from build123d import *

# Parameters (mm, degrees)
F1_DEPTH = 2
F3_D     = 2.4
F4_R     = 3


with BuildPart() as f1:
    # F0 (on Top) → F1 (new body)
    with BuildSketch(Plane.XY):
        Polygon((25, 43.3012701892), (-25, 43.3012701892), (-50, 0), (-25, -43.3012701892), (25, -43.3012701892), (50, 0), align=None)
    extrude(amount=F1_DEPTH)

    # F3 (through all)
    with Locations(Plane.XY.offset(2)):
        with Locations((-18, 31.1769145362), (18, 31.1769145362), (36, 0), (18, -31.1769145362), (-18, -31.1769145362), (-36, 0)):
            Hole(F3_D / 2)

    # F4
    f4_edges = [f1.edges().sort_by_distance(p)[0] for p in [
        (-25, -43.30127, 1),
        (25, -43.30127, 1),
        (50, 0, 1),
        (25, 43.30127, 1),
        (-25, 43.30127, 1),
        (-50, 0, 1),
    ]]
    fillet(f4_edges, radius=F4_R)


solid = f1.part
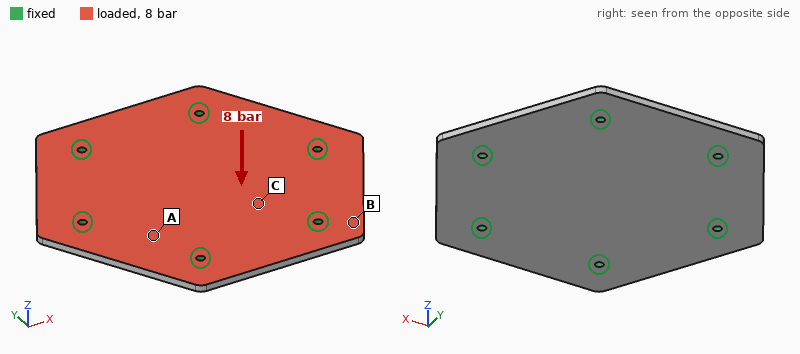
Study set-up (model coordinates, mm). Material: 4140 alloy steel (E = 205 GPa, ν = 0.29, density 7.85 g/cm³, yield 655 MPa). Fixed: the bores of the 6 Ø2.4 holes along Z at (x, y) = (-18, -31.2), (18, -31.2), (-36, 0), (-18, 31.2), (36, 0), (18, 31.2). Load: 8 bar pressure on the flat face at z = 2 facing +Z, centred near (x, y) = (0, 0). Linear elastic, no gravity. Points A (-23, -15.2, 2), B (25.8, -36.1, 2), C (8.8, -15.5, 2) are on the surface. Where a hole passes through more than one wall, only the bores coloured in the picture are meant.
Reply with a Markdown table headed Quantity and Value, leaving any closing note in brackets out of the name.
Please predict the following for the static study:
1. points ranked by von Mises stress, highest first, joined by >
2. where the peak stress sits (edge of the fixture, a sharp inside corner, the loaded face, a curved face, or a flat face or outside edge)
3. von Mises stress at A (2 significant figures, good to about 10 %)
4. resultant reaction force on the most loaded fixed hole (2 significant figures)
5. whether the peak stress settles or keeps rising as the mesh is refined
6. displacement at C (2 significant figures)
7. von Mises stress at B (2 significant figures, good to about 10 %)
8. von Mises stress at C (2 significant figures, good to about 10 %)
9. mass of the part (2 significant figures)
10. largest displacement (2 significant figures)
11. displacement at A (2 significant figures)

| Quantity | Value |
|---|---|
| points ranked by von Mises stress, highest first, joined by > | A > C > B |
| where the peak stress sits | edge of the fixture |
| von Mises stress at A | 120 MPa |
| resultant reaction force on the most loaded fixed hole | 860 N |
| whether the peak stress settles or keeps rising as the mesh is refined | keeps rising |
| displacement at C | 0.12 mm |
| von Mises stress at B | 34 MPa |
| von Mises stress at C | 74 MPa |
| mass of the part | 100 g |
| largest displacement | 0.19 mm |
| displacement at A | 0.062 mm |
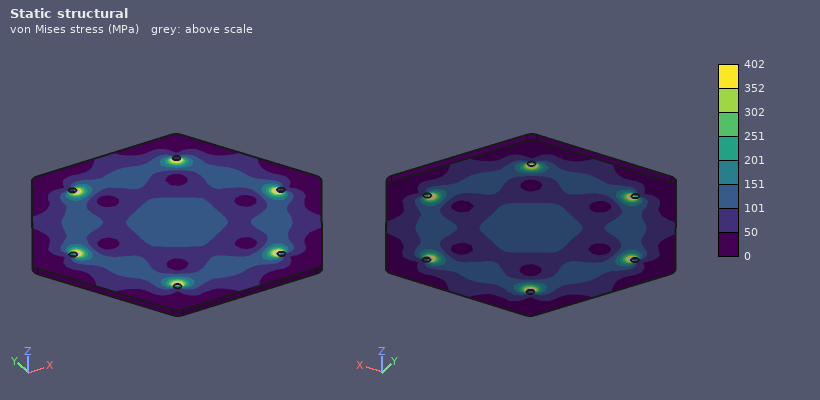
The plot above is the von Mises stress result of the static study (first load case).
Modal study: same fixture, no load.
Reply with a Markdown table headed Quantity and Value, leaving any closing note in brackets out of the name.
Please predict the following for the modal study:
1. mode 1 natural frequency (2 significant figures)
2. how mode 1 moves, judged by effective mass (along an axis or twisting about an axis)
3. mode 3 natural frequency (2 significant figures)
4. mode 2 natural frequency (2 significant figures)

| Quantity | Value |
|---|---|
| mode 1 natural frequency | 3100 Hz |
| how mode 1 moves, judged by effective mass | along Z |
| mode 3 natural frequency | 6300 Hz |
| mode 2 natural frequency | 5900 Hz |
